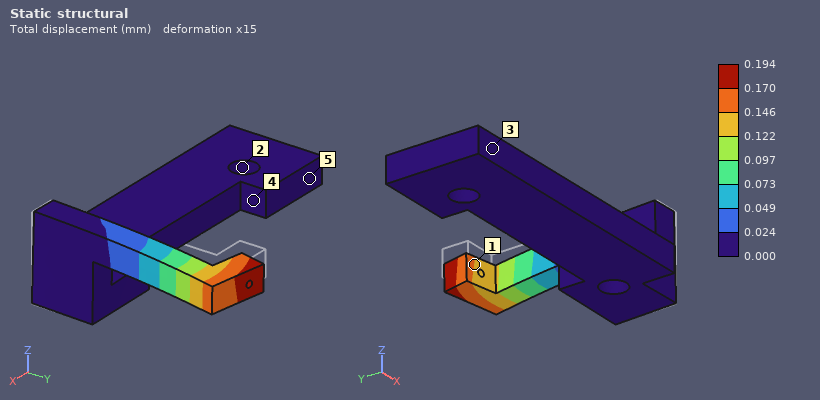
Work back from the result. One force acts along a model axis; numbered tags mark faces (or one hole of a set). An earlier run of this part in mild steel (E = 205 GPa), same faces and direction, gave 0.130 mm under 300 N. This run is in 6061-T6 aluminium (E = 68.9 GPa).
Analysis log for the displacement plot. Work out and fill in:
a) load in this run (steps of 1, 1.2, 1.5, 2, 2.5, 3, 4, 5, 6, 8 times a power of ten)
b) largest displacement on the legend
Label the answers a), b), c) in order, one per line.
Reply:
a) 150 N
b) 0.194 mm
